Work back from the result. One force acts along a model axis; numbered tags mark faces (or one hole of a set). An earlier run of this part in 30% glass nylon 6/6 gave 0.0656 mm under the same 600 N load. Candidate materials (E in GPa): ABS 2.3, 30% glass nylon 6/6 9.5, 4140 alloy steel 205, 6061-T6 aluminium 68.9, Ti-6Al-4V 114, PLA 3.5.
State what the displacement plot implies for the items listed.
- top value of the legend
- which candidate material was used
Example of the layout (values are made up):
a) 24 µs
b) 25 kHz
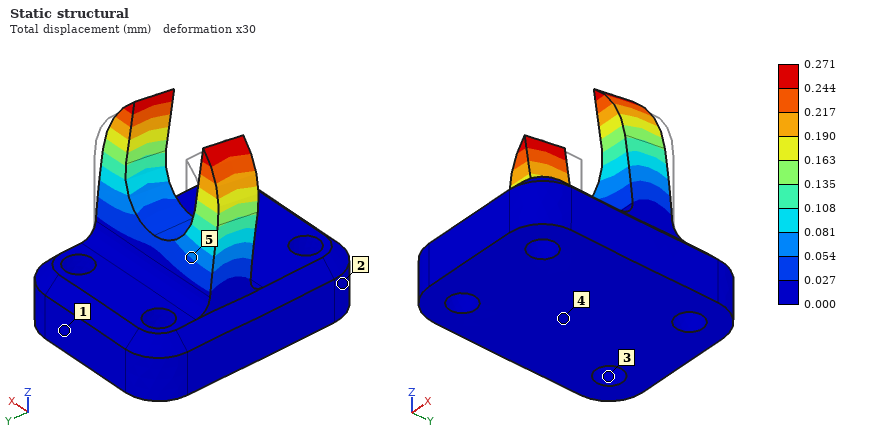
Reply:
a) 0.271 mm
b) ABS
